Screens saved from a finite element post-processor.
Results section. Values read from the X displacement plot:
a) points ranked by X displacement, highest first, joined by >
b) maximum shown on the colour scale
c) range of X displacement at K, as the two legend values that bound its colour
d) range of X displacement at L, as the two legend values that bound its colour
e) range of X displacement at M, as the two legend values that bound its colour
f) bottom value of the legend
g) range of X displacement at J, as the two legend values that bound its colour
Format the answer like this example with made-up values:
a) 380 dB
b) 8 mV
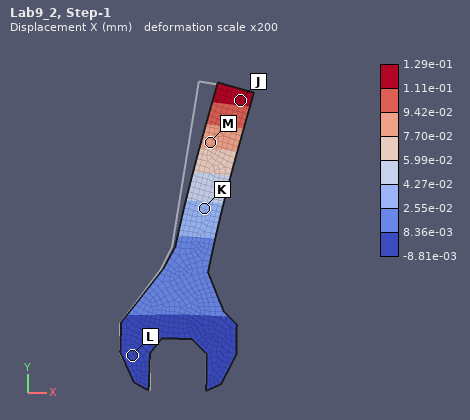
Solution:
a) J > M > K > L
b) 1.29e-01 mm
c) 2.55e-02 to 4.27e-02 mm
d) -8.81e-03 to 8.36e-03 mm
e) 7.70e-02 to 9.42e-02 mm
f) -8.81e-03 mm
g) 1.11e-01 to 1.29e-01 mm
